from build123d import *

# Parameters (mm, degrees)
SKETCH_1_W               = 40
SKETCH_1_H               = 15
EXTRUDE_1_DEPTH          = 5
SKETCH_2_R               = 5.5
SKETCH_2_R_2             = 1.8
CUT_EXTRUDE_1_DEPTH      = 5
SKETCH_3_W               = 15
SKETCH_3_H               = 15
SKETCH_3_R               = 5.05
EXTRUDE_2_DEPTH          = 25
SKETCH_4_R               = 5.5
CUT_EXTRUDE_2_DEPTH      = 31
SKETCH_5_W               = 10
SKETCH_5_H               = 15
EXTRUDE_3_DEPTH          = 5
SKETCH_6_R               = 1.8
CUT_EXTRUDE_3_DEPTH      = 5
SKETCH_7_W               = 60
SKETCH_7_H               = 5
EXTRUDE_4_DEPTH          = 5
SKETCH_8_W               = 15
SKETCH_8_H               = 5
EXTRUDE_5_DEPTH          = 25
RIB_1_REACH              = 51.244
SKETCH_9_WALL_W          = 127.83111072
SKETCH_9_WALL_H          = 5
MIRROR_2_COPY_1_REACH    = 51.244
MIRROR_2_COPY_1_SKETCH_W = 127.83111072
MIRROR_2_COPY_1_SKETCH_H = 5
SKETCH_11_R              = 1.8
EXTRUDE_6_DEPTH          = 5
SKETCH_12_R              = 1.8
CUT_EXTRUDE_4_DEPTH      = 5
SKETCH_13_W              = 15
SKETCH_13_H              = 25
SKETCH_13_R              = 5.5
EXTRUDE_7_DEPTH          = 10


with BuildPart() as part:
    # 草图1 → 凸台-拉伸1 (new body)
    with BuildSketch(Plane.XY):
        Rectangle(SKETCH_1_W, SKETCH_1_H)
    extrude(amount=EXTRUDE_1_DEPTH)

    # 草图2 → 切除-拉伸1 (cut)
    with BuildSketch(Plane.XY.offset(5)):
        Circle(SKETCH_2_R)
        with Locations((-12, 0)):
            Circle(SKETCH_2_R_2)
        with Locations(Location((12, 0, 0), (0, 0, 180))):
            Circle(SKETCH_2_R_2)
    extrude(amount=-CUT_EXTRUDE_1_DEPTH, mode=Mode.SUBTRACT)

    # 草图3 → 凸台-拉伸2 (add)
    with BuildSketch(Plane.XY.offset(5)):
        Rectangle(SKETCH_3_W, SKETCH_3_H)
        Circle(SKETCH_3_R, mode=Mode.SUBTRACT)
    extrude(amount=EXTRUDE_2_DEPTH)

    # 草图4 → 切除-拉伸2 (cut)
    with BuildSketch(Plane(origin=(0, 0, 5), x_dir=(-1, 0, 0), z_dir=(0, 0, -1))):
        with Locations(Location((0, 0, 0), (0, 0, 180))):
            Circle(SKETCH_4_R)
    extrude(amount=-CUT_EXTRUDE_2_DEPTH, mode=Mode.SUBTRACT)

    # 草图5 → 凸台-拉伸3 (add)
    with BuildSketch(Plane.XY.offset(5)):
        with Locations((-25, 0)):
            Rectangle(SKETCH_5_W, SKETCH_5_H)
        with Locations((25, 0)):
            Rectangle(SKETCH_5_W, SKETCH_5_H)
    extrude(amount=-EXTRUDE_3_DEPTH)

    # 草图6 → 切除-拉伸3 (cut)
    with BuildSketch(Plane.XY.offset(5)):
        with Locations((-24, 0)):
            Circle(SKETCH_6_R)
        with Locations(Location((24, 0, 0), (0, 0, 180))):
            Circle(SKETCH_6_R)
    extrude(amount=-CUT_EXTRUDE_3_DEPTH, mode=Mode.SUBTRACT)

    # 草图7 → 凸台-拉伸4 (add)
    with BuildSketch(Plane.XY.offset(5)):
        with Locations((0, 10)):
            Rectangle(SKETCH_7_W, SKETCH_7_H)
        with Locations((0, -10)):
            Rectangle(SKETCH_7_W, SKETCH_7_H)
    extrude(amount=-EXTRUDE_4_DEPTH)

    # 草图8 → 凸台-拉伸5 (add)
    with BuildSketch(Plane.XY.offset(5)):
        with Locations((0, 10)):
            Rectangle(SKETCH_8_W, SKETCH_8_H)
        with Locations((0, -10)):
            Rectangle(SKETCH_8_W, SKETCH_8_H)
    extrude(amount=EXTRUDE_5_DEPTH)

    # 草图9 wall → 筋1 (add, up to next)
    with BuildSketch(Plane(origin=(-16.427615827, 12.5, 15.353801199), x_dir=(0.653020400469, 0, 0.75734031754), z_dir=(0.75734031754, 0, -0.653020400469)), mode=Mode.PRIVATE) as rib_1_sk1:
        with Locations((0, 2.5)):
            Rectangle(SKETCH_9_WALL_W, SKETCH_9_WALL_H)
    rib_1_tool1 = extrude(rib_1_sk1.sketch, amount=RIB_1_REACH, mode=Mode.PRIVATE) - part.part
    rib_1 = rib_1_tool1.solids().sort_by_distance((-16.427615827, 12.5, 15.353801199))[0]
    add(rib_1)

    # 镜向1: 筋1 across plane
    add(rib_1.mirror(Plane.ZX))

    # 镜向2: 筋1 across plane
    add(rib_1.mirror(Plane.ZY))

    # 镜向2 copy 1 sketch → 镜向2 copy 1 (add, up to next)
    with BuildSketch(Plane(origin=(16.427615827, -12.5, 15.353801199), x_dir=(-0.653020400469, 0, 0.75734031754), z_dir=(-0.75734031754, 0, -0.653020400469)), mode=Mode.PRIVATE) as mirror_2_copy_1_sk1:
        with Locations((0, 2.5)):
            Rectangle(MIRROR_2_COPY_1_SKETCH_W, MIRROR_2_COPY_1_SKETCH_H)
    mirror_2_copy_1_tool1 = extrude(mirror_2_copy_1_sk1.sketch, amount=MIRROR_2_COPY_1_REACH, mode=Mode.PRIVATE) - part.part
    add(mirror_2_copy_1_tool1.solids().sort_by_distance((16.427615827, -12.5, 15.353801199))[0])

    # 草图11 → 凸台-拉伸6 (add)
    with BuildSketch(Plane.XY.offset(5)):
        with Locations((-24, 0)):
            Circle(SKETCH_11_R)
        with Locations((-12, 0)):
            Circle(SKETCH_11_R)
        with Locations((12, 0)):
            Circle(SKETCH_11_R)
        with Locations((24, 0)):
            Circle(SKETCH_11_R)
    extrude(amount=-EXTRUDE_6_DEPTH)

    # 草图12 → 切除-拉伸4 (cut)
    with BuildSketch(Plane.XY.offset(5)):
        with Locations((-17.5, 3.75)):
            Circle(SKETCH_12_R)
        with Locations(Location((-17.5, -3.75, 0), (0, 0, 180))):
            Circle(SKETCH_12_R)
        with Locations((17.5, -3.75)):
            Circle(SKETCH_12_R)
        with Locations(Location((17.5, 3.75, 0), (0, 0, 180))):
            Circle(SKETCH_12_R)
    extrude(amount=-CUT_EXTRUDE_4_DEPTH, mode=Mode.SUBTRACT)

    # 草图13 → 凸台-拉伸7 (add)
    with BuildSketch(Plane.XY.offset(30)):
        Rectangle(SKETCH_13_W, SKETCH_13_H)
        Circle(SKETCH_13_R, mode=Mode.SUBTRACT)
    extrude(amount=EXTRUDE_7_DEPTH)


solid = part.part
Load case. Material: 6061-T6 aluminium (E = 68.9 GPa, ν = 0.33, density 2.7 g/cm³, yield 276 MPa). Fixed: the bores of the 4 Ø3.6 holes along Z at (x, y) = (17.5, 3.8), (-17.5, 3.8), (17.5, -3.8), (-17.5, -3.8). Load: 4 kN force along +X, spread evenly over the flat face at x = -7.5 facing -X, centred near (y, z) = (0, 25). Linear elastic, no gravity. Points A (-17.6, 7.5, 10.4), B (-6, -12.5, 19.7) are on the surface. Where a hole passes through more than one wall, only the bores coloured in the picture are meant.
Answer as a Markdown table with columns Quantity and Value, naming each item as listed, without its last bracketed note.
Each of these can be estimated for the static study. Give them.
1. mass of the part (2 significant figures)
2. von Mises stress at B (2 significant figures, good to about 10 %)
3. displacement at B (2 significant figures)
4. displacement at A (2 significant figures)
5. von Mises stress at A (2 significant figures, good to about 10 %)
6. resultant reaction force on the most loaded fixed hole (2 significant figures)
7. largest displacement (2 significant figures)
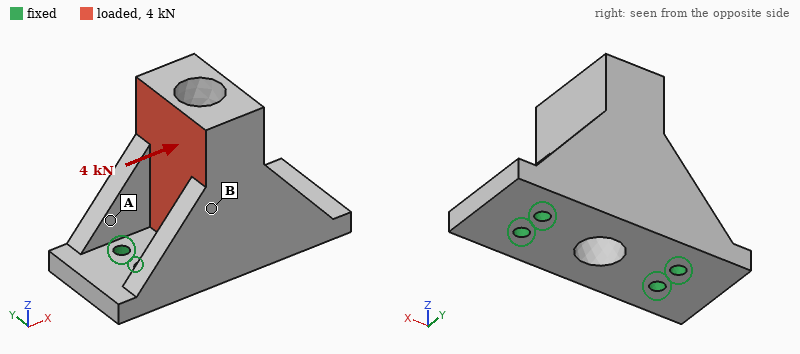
| Quantity | Value |
|---|---|
| mass of the part | 55 g |
| von Mises stress at B | 19 MPa |
| displacement at B | 15 µm |
| displacement at A | 12 µm |
| von Mises stress at A | 39 MPa |
| resultant reaction force on the most loaded fixed hole | 1.6 kN |
| largest displacement | 50 µm |
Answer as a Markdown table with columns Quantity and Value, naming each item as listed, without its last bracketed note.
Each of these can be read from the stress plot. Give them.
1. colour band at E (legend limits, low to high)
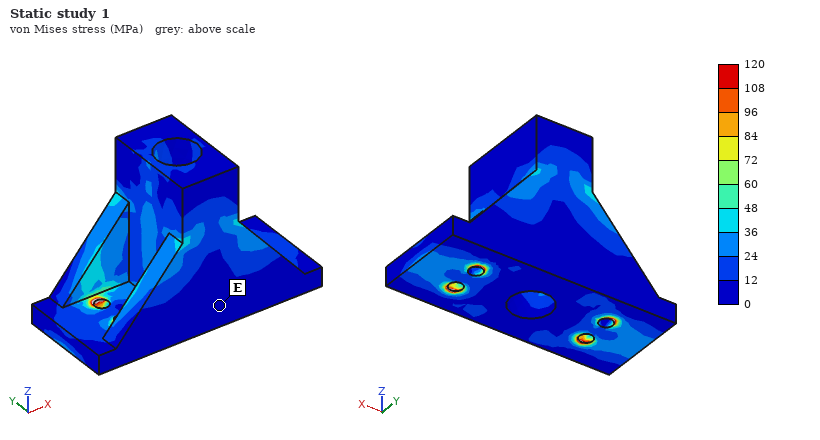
| Quantity | Value |
|---|---|
| colour band at E | 0 to 12 MPa |
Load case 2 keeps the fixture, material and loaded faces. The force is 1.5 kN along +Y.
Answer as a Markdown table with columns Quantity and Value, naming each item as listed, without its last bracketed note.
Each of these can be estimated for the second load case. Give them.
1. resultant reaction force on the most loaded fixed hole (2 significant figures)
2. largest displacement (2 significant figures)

| Quantity | Value |
|---|---|
| resultant reaction force on the most loaded fixed hole | 1.4 kN |
| largest displacement | 73 µm |
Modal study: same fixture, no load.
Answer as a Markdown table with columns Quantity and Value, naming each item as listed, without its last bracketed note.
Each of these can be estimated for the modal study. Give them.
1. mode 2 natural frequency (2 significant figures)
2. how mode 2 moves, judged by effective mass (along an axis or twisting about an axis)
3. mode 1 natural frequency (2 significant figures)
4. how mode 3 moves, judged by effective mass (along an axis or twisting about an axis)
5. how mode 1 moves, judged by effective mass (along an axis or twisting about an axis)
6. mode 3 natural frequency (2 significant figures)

| Quantity | Value |
|---|---|
| mode 2 natural frequency | 11 kHz |
| how mode 2 moves, judged by effective mass | along X |
| mode 1 natural frequency | 5300 Hz |
| how mode 3 moves, judged by effective mass | along Z |
| how mode 1 moves, judged by effective mass | along Y |
| mode 3 natural frequency | 15 kHz |
